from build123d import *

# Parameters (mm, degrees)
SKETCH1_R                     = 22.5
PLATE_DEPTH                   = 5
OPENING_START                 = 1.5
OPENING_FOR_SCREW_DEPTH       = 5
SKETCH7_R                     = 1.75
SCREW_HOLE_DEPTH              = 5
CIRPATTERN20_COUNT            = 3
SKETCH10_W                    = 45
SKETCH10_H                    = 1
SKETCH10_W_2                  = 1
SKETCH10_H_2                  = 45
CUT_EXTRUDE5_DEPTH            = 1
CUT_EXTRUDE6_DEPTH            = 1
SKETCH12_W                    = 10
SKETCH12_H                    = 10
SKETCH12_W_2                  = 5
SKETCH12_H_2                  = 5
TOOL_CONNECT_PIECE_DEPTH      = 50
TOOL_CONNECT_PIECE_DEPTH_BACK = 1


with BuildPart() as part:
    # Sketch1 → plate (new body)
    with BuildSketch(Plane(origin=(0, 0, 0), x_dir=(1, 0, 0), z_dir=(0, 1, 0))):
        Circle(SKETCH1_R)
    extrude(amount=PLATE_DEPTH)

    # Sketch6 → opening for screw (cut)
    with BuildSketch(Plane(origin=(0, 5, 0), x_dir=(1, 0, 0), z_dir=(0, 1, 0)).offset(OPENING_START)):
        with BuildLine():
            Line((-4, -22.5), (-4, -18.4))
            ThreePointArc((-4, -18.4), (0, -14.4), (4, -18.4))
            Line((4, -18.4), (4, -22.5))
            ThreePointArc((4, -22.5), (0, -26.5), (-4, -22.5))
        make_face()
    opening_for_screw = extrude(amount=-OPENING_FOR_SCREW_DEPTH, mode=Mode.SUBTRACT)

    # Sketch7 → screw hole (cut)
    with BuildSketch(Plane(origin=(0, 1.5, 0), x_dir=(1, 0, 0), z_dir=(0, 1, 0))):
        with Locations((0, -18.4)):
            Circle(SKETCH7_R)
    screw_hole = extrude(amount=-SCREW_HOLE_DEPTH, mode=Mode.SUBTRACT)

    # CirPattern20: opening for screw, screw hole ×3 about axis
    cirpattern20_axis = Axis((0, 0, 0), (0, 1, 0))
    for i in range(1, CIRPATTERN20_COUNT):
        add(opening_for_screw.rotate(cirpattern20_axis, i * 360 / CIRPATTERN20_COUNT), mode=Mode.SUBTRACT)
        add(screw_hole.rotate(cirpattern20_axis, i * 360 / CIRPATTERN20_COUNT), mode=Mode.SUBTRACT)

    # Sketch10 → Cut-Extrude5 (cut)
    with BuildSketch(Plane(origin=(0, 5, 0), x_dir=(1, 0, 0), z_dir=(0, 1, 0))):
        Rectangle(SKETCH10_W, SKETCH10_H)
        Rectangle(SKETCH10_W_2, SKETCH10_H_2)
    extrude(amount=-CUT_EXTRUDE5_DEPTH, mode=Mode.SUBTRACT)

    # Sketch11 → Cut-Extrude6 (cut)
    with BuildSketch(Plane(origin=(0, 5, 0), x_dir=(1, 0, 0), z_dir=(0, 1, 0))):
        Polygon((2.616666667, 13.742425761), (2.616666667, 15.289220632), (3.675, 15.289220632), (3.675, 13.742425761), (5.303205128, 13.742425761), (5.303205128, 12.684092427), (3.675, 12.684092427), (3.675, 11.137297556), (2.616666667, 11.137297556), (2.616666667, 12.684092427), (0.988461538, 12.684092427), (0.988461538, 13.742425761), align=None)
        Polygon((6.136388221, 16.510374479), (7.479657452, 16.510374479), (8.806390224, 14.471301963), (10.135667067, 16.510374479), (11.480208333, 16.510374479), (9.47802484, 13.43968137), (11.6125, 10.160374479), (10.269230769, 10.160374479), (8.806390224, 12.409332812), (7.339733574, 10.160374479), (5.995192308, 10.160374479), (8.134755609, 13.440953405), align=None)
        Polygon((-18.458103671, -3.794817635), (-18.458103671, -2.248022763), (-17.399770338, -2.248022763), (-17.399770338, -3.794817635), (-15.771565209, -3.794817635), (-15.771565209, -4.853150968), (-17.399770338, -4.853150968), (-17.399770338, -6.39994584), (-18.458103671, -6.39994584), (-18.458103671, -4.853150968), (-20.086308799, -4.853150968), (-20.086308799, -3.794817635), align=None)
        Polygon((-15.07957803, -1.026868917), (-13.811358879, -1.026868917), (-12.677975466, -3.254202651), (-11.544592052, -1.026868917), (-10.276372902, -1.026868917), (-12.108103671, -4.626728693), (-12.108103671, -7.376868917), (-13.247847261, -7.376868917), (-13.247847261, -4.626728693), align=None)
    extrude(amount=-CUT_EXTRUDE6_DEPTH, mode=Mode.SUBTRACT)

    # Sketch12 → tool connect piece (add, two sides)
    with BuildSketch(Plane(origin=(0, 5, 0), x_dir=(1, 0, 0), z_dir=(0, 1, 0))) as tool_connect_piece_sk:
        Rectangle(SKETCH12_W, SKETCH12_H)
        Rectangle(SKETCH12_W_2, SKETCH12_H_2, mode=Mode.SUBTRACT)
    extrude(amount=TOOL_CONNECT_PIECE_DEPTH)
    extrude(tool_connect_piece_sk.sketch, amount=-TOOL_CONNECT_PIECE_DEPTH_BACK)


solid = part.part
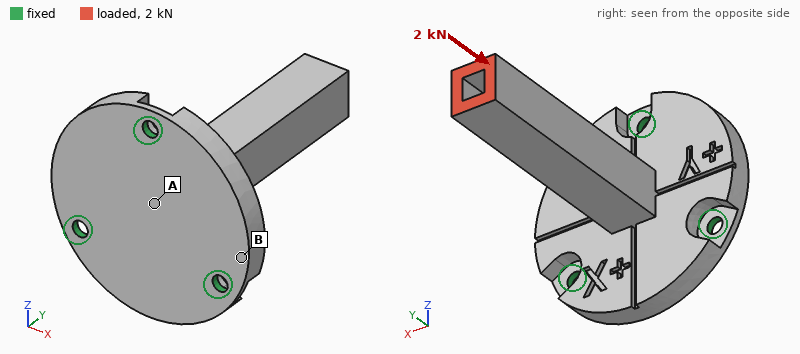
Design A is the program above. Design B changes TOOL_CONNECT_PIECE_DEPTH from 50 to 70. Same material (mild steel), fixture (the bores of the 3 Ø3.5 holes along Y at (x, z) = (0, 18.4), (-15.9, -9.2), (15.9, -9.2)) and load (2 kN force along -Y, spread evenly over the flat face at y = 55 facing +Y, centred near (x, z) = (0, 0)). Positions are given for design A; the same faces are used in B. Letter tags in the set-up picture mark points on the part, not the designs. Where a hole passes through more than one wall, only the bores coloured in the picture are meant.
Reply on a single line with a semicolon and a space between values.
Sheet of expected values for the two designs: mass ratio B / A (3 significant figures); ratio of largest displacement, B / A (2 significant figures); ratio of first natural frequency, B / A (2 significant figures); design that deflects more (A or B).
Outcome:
1.14; 1.1; 0.56; B
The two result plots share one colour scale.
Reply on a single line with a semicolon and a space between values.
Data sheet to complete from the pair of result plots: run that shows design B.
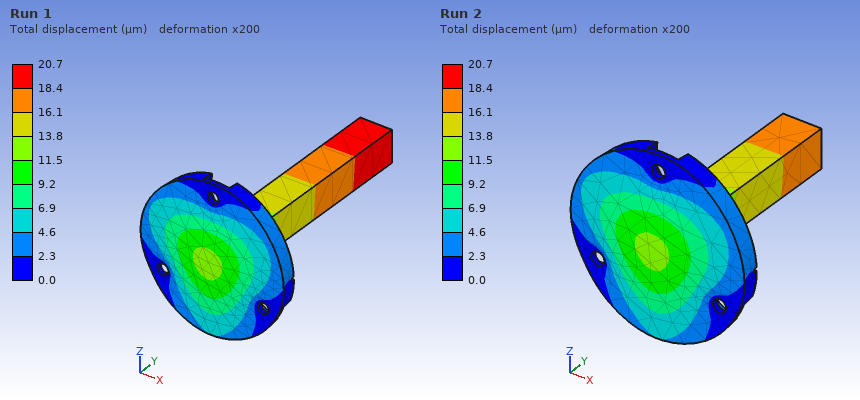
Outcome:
Run 1
